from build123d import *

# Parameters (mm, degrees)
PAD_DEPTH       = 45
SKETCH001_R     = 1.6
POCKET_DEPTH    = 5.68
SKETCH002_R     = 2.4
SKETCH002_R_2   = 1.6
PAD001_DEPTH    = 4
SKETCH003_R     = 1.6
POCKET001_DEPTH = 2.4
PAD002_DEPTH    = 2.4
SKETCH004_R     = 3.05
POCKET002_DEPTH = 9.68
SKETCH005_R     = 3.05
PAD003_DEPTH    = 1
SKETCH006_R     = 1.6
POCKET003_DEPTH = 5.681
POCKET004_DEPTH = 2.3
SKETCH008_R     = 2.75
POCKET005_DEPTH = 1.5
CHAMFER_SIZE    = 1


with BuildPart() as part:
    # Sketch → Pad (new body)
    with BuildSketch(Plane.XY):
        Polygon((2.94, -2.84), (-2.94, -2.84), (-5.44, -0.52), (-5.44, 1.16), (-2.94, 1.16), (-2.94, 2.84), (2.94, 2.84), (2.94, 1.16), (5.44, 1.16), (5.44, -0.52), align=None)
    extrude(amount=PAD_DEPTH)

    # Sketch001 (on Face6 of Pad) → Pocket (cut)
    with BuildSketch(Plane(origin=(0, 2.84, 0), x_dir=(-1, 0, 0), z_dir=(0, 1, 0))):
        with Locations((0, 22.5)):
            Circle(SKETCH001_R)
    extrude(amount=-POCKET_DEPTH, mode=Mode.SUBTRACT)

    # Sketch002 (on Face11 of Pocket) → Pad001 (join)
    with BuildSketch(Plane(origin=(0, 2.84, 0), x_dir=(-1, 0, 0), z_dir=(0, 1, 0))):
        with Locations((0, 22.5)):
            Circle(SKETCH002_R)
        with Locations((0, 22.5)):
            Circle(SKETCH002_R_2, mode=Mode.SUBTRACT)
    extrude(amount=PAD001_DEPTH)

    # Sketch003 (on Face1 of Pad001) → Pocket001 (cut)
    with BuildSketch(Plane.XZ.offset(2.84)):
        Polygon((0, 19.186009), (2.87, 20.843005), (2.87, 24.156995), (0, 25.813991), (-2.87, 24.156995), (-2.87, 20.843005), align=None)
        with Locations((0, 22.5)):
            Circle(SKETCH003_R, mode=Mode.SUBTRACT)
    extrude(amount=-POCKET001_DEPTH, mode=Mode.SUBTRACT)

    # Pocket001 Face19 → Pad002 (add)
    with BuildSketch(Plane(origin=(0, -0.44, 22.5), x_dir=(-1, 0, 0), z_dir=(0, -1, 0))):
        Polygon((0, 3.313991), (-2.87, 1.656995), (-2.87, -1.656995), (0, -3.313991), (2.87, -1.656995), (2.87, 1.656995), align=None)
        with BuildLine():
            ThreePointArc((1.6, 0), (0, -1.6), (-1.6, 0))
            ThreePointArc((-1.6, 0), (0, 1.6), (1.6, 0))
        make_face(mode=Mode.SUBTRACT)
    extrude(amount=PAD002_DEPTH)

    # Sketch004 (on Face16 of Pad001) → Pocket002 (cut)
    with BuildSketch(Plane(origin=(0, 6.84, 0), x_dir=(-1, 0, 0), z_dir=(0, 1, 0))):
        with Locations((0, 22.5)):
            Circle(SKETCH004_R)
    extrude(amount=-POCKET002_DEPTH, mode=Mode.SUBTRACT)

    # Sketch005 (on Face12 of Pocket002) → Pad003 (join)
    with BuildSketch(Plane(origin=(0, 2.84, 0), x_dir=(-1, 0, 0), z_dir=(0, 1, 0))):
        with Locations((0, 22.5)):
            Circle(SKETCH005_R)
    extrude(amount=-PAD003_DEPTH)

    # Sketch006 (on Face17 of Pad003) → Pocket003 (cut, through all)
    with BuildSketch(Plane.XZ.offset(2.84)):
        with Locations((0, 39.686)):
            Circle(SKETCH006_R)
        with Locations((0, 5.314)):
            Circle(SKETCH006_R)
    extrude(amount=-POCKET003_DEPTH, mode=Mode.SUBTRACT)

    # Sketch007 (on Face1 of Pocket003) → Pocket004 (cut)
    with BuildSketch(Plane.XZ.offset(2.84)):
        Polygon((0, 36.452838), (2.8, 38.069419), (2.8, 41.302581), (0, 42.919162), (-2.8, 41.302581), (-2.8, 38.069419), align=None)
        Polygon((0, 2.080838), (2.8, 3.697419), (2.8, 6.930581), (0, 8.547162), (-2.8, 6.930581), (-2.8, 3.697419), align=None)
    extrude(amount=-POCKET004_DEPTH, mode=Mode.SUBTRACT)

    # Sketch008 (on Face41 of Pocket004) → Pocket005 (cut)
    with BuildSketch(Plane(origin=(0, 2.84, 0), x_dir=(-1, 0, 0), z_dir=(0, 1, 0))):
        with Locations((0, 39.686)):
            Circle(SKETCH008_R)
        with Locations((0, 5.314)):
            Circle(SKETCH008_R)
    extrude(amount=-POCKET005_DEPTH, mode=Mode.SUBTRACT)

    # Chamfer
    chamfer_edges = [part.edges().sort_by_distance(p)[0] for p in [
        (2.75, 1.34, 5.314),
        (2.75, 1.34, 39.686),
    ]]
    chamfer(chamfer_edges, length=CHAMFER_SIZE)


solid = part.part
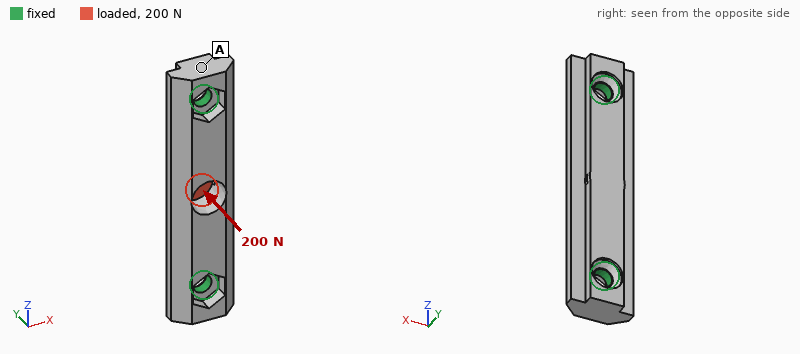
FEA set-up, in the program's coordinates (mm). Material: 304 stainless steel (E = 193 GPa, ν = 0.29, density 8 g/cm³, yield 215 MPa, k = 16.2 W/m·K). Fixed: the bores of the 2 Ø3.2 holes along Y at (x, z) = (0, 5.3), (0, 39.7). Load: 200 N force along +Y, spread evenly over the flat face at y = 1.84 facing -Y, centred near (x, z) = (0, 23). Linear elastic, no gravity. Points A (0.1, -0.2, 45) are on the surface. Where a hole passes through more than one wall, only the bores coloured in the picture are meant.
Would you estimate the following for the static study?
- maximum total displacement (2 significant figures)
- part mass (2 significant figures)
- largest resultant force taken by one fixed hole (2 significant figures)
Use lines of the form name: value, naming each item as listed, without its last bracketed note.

maximum total displacement: 7.7 µm
part mass: 14 g
largest resultant force taken by one fixed hole: 100 N
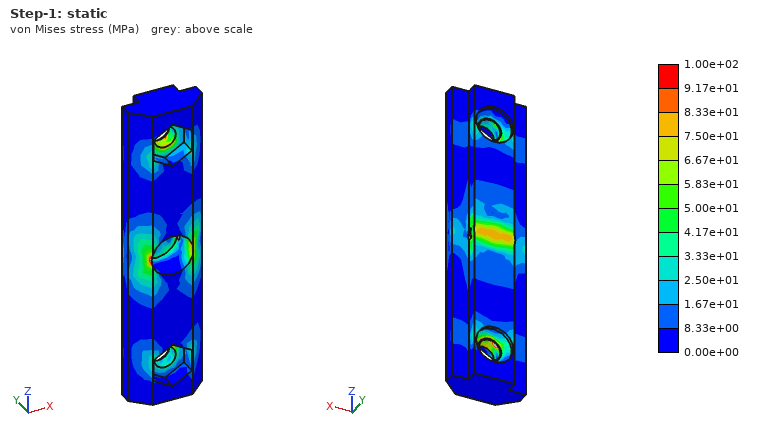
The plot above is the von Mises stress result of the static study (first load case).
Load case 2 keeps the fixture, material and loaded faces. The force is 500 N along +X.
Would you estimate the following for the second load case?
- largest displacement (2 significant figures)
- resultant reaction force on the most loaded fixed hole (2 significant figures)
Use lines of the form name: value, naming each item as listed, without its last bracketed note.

largest displacement: 7.6 µm
resultant reaction force on the most loaded fixed hole: 250 N
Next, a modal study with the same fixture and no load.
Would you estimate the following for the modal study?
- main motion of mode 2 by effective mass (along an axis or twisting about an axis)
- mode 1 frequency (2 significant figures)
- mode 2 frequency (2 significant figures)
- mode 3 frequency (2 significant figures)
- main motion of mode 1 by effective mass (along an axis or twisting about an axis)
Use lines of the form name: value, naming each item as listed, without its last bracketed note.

main motion of mode 2 by effective mass: along X
mode 1 frequency: 13 kHz
mode 2 frequency: 22 kHz
mode 3 frequency: 25 kHz
main motion of mode 1 by effective mass: along Y
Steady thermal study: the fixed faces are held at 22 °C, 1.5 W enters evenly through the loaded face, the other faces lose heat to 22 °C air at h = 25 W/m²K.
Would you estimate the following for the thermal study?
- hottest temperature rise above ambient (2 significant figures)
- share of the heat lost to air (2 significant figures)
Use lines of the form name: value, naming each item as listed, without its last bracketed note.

hottest temperature rise above ambient: 30 K
share of the heat lost to air: 18 %
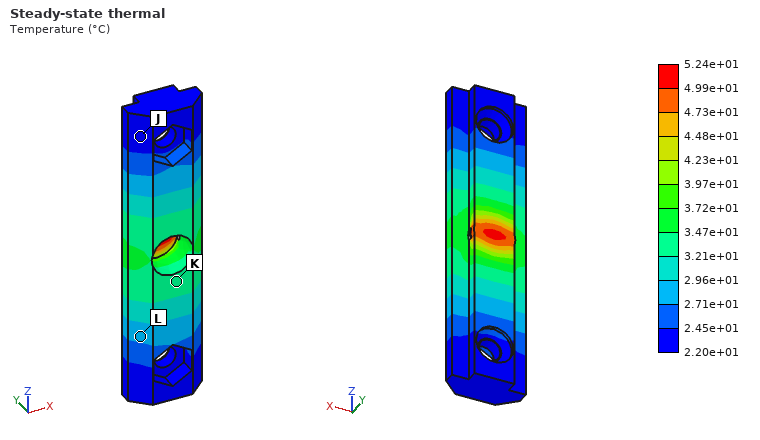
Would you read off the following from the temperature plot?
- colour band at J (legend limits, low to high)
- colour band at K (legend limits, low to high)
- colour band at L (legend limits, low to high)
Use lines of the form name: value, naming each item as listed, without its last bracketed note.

colour band at J: 2.20e+01 to 2.45e+01 °C
colour band at K: 3.21e+01 to 3.47e+01 °C
colour band at L: 2.71e+01 to 2.96e+01 °C
